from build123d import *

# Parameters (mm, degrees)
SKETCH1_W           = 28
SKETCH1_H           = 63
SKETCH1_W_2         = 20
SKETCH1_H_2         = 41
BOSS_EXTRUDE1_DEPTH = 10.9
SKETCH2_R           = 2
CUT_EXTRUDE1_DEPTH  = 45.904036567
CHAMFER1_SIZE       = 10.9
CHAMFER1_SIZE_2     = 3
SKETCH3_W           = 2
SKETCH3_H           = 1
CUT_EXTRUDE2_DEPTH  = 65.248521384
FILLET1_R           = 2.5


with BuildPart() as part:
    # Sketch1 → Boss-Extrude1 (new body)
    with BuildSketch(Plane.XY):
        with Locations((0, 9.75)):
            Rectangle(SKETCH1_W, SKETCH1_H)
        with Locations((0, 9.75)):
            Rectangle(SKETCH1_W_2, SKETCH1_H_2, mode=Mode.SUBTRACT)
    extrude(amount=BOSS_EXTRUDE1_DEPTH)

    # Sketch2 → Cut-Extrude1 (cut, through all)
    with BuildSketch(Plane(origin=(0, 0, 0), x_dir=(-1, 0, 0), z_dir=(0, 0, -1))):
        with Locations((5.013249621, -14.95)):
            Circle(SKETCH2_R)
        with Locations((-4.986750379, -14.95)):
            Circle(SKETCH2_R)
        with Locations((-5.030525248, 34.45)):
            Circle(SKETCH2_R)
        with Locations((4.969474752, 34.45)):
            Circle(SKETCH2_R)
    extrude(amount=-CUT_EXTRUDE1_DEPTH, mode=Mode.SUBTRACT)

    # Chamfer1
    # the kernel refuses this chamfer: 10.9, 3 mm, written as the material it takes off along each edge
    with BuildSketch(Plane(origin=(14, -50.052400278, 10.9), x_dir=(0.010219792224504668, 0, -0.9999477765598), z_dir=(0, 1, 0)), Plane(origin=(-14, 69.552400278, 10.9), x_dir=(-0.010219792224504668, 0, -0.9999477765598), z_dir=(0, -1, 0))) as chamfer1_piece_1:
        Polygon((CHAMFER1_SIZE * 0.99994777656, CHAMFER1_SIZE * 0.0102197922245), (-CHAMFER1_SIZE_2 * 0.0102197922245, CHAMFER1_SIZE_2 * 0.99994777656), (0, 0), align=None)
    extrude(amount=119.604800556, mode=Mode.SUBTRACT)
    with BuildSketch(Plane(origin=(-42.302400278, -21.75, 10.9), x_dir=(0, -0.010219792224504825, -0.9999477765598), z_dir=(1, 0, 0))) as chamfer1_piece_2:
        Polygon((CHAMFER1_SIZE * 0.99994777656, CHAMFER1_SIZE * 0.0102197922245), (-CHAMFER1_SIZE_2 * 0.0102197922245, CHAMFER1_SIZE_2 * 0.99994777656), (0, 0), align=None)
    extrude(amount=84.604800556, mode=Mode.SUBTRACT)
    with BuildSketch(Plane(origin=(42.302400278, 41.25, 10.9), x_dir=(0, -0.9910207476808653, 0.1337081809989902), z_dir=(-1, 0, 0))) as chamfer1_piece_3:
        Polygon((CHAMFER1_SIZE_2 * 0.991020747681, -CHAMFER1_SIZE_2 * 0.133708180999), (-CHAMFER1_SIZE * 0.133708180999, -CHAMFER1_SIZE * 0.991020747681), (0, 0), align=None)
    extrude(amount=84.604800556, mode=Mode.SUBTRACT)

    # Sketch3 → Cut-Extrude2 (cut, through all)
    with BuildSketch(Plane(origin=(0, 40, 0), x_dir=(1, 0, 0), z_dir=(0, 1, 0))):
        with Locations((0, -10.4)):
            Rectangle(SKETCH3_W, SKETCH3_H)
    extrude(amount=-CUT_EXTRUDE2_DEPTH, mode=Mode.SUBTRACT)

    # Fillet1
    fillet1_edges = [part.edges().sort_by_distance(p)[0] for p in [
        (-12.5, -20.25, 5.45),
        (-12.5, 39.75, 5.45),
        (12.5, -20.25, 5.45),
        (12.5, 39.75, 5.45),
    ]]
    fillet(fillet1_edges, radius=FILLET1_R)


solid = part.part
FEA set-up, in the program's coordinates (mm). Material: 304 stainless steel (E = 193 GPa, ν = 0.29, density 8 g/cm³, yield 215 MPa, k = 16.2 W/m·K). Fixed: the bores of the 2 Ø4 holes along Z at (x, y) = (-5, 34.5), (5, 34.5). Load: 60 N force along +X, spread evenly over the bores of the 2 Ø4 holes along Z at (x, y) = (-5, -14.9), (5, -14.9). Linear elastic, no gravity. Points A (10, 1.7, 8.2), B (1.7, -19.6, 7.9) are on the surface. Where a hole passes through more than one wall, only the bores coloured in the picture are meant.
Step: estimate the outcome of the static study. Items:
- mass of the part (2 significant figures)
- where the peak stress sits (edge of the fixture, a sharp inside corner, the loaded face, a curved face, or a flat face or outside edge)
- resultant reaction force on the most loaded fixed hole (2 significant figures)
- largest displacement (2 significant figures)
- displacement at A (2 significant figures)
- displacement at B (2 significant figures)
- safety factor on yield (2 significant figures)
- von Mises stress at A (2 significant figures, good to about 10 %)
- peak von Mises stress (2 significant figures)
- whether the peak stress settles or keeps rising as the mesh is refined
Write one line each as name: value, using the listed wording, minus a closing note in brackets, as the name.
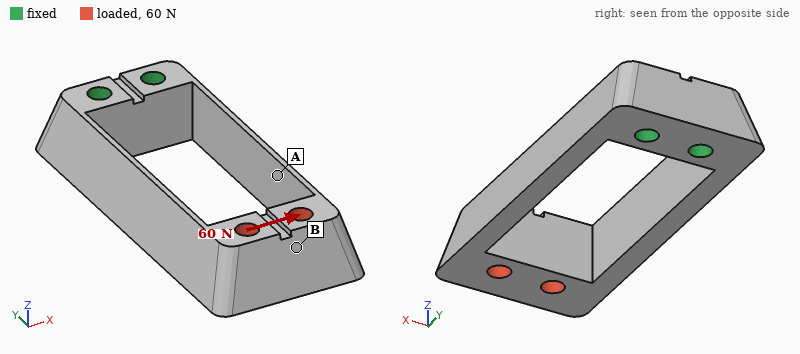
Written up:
mass of the part: 54 g
where the peak stress sits: a flat face or outside edge
resultant reaction force on the most loaded fixed hole: 140 N
largest displacement: 62 µm
displacement at A: 44 µm
displacement at B: 59 µm
safety factor on yield: 3.6
von Mises stress at A: 14 MPa
peak von Mises stress: 59 MPa
whether the peak stress settles or keeps rising as the mesh is refined: settles
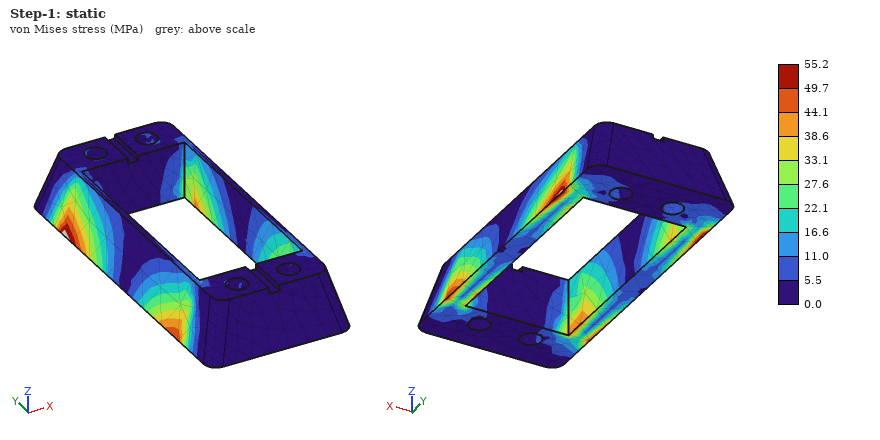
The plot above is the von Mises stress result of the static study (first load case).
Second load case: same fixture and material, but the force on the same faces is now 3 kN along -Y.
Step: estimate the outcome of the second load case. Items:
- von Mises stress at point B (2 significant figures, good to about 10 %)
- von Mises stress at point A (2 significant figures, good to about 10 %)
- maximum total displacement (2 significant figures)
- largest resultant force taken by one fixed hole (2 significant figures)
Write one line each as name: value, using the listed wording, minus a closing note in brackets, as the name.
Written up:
von Mises stress at point B: 68 MPa
von Mises stress at point A: 88 MPa
maximum total displacement: 53 µm
largest resultant force taken by one fixed hole: 1.5 kN
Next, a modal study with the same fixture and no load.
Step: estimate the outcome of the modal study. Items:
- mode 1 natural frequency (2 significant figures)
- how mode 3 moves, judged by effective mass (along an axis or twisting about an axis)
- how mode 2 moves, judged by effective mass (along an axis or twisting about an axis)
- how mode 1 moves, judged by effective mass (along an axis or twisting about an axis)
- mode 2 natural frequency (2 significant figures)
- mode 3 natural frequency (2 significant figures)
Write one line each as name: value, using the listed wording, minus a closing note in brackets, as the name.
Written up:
mode 1 natural frequency: 1000 Hz
how mode 3 moves, judged by effective mass: twisting about Y
how mode 2 moves, judged by effective mass: along Z
how mode 1 moves, judged by effective mass: along X
mode 2 natural frequency: 1500 Hz
mode 3 natural frequency: 3700 Hz
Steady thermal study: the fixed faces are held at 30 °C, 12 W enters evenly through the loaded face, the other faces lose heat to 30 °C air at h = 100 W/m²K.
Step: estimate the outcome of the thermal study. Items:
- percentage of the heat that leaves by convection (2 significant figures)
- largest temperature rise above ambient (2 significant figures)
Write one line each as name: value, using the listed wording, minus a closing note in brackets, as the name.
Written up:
percentage of the heat that leaves by convection: 98 %
largest temperature rise above ambient: 83 K
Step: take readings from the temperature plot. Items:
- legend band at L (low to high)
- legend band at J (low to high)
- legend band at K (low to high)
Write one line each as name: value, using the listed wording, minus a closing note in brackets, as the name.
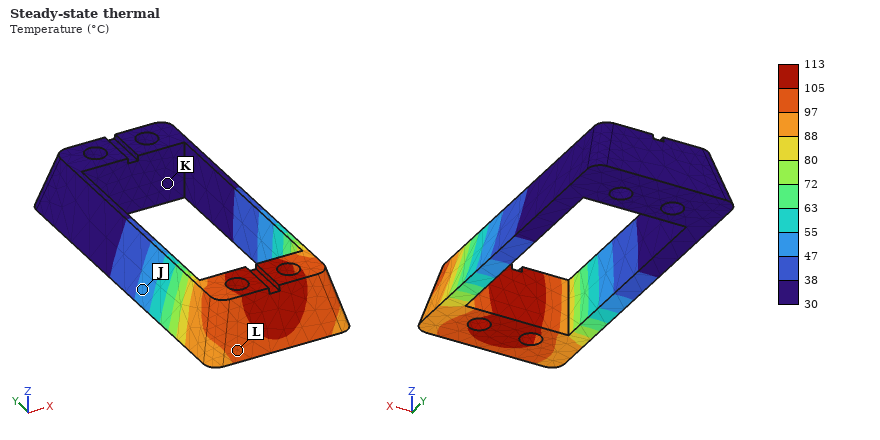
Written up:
legend band at L: 97 to 105 °C
legend band at J: 47 to 55 °C
legend band at K: 30 to 38 °C
